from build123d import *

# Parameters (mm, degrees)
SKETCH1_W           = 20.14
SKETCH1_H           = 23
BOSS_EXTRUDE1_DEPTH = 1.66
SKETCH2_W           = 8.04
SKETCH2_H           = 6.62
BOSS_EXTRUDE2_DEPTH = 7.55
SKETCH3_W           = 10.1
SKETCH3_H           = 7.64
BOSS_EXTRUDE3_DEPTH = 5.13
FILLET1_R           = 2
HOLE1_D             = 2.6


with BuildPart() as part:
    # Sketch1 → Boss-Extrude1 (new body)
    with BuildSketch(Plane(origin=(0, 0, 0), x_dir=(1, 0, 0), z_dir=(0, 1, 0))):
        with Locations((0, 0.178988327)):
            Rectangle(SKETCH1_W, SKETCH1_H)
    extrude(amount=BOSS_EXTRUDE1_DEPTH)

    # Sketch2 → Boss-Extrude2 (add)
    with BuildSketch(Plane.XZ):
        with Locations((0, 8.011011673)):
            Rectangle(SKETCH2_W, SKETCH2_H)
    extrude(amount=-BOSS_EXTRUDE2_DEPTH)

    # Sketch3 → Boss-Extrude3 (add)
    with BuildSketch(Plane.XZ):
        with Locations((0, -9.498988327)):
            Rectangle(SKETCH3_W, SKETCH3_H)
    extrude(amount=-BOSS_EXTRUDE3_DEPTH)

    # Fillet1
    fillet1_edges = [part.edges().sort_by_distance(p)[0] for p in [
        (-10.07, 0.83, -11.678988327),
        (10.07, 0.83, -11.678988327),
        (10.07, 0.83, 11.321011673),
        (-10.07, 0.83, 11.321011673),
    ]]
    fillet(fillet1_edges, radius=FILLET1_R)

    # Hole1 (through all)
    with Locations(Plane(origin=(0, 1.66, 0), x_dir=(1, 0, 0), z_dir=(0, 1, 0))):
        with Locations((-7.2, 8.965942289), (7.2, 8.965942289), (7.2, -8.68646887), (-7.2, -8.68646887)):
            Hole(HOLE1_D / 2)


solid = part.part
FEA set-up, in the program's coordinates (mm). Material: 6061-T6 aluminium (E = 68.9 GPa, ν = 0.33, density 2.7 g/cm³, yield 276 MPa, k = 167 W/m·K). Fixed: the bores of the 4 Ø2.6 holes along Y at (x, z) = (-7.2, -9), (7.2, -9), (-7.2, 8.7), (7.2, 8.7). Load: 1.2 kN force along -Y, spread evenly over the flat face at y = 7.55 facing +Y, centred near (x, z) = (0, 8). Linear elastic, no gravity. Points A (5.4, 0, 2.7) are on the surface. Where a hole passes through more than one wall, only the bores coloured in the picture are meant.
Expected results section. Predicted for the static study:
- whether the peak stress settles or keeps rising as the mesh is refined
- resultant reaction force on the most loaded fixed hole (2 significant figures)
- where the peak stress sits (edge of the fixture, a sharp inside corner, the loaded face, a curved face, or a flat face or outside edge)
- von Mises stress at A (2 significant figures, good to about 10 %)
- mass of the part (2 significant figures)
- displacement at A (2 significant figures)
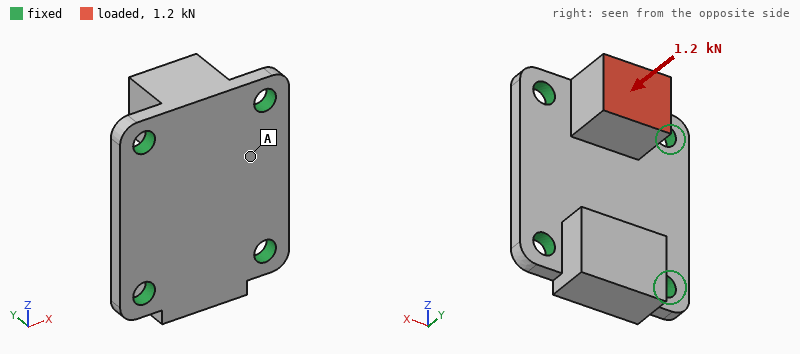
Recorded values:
keeps rising
620 N
edge of the fixture
35 MPa
3.6 g
10.0 µm
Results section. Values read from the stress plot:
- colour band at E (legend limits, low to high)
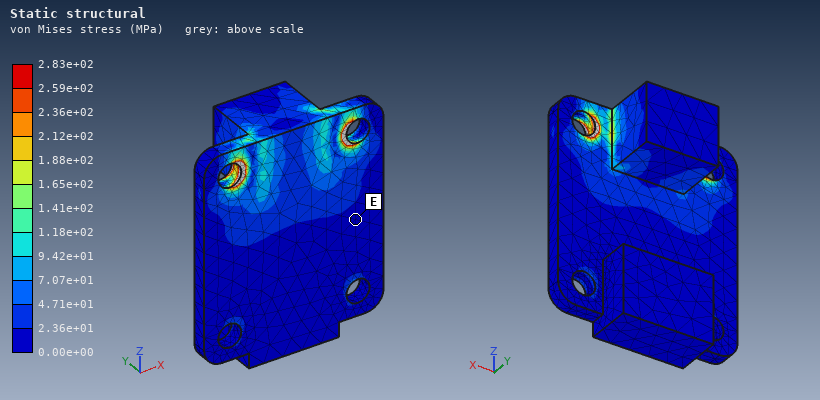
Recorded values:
0.00e+00 to 2.36e+01 MPa
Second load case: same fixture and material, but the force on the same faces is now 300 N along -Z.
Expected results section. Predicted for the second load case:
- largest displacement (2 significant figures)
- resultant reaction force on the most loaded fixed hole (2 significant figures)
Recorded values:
38 µm
120 N
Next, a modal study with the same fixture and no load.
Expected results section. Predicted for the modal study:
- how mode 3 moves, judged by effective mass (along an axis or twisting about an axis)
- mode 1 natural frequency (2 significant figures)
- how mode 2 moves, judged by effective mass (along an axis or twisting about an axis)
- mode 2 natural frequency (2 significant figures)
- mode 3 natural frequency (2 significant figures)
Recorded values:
twisting about Z
20 kHz
along Z
30 kHz
37 kHz
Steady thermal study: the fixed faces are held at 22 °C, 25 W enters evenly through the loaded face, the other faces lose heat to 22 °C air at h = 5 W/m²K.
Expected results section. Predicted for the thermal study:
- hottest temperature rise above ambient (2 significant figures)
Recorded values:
37 K
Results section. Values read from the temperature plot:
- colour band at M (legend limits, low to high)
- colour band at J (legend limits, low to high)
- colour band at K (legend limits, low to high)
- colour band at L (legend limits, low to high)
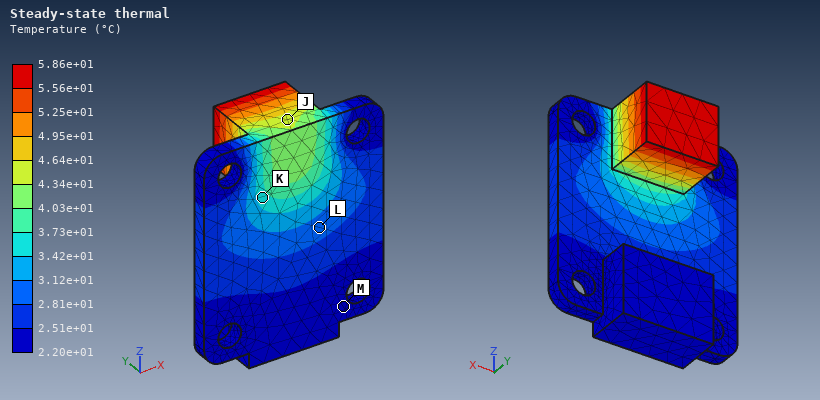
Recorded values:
2.20e+01 to 2.51e+01 °C
4.34e+01 to 4.64e+01 °C
3.42e+01 to 3.73e+01 °C
2.81e+01 to 3.12e+01 °C
